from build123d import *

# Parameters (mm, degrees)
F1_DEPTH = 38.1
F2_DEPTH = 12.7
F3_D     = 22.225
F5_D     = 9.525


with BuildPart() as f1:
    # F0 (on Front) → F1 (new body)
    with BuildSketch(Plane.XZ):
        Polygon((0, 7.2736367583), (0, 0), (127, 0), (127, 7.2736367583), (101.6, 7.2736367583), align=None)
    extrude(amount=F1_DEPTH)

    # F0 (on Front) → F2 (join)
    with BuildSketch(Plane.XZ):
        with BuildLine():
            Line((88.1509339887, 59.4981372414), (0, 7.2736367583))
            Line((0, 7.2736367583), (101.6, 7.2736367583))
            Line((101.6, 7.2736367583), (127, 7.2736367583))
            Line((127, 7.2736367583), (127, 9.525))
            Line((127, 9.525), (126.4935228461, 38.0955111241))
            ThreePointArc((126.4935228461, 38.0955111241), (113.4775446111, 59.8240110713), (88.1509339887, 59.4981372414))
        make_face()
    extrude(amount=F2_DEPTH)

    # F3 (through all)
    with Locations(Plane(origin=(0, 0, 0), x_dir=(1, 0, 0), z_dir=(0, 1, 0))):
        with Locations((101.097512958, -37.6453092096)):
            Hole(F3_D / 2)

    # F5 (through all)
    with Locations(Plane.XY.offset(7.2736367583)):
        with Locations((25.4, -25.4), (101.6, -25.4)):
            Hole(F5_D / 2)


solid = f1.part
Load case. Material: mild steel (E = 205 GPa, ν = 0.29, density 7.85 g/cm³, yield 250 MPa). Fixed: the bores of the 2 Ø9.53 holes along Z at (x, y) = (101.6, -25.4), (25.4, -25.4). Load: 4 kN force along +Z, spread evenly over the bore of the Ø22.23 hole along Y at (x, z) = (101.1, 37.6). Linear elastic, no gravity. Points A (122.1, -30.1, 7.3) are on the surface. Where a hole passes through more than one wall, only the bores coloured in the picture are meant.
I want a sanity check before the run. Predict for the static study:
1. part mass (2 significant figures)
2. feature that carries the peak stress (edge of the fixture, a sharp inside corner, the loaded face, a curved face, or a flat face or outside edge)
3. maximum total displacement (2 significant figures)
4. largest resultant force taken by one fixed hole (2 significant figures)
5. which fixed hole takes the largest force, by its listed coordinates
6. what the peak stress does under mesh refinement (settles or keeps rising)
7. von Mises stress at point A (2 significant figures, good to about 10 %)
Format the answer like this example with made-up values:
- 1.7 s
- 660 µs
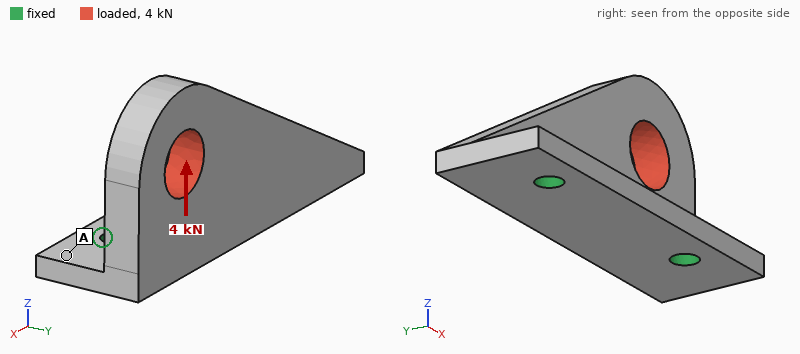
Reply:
- 660 g
- edge of the fixture
- 80 µm
- 3.9 kN
- (101.6, -25.4)
- keeps rising
- 24 MPa
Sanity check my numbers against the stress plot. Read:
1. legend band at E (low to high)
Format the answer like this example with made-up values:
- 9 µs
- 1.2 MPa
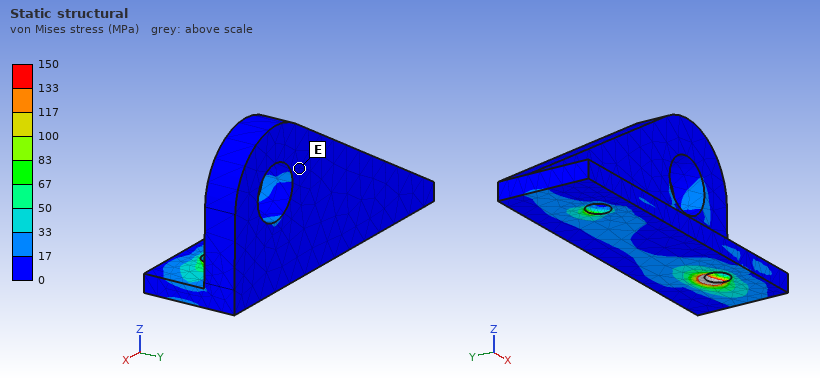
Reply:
- 0 to 17 MPa
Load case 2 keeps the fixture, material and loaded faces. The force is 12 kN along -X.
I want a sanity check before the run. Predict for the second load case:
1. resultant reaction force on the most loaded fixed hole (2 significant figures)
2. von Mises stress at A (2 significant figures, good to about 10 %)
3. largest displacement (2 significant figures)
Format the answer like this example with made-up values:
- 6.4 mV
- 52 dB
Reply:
- 8.4 kN
- 26 MPa
- 63 µm
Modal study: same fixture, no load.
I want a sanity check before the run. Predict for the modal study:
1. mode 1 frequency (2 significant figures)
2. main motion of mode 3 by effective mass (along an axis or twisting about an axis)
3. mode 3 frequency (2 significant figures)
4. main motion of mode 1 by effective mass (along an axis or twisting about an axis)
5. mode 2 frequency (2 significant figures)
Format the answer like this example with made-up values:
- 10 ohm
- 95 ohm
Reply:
- 1600 Hz
- along Z
- 5500 Hz
- along Y
- 4300 Hz
